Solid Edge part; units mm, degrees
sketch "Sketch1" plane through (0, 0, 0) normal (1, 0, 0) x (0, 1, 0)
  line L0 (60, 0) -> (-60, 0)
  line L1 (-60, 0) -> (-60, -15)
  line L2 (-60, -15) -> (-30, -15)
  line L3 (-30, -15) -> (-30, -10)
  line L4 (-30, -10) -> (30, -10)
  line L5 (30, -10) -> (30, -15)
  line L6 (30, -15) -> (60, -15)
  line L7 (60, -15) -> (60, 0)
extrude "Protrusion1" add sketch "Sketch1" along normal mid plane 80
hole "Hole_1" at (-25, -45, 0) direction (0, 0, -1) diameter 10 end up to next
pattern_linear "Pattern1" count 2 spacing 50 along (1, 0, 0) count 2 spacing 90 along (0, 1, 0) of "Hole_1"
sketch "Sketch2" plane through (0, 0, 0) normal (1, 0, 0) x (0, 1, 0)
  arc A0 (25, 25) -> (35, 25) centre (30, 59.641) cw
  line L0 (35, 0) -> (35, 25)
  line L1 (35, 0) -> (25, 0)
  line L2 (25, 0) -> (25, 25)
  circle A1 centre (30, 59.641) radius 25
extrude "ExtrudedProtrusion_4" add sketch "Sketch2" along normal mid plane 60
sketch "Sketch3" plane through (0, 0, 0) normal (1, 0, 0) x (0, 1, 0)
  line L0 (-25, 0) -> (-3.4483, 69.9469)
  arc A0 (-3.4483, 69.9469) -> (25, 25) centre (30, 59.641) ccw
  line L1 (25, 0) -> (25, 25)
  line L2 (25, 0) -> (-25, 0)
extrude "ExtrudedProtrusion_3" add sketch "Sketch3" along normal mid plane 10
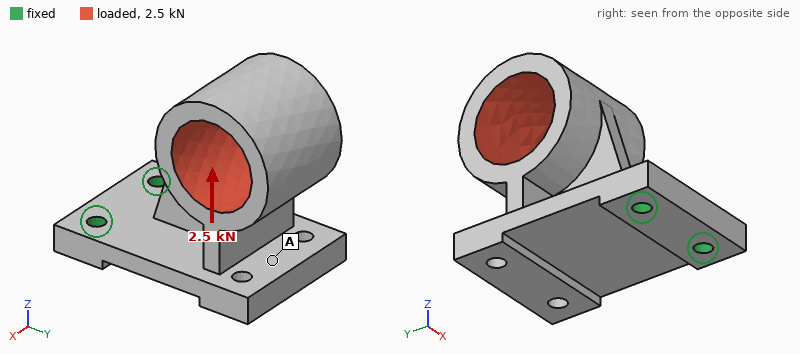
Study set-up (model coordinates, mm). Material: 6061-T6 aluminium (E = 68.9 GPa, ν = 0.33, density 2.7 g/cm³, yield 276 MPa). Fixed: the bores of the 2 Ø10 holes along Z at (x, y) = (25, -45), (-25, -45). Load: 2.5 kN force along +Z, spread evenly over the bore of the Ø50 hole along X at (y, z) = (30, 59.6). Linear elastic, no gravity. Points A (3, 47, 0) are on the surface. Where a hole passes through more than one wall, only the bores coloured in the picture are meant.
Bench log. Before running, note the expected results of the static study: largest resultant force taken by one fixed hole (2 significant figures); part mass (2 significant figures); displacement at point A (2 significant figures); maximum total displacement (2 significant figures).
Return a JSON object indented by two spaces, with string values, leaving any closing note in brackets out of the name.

{
  "largest resultant force taken by one fixed hole": "1.3 kN",
  "part mass": "700 g",
  "displacement at point A": "0.55 mm",
  "maximum total displacement": "0.91 mm"
}
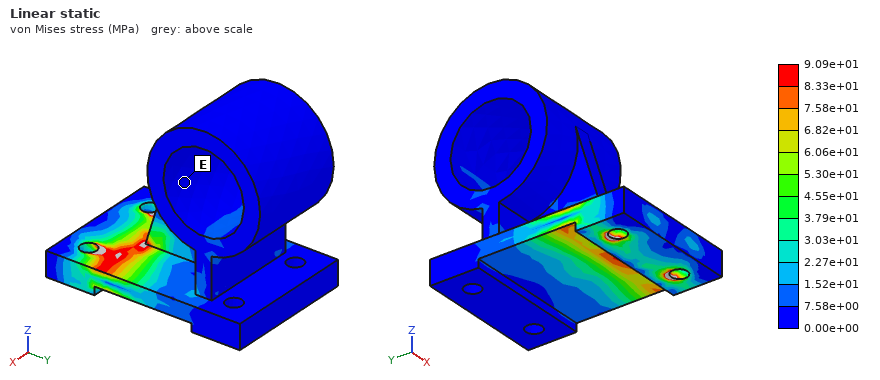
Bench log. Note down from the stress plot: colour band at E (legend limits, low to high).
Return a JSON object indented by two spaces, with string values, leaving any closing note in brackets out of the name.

{
  "colour band at E": "0.00e+00 to 7.58e+00 MPa"
}
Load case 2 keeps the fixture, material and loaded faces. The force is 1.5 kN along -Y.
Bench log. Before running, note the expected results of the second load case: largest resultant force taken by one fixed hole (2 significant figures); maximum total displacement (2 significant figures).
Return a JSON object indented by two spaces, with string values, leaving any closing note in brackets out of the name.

{
  "largest resultant force taken by one fixed hole": "830 N",
  "maximum total displacement": "0.65 mm"
}
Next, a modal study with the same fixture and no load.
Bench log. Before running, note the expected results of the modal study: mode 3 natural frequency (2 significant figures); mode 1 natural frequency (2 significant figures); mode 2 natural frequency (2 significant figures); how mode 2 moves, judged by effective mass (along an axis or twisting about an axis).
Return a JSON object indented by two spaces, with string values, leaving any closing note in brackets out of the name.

{
  "mode 3 natural frequency": "2300 Hz",
  "mode 1 natural frequency": "380 Hz",
  "mode 2 natural frequency": "590 Hz",
  "how mode 2 moves, judged by effective mass": "along X"
}
